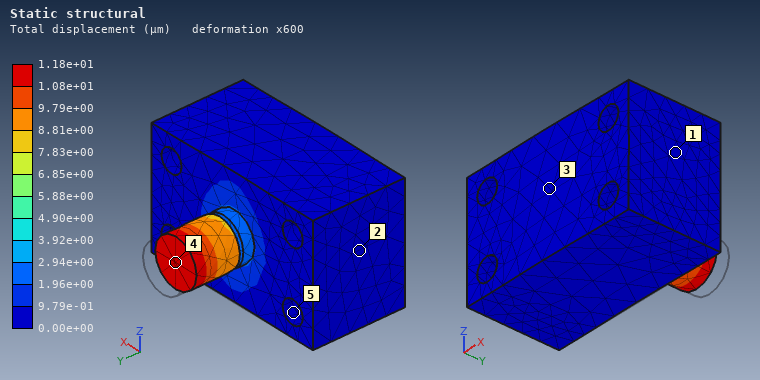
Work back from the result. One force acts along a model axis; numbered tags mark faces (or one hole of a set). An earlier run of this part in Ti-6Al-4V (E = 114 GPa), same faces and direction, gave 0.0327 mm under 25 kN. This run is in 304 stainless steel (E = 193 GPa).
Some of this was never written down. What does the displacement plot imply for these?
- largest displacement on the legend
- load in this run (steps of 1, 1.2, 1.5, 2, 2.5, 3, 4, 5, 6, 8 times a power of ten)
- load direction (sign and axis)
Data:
1.18e+01 µm
15 kN
-Y
